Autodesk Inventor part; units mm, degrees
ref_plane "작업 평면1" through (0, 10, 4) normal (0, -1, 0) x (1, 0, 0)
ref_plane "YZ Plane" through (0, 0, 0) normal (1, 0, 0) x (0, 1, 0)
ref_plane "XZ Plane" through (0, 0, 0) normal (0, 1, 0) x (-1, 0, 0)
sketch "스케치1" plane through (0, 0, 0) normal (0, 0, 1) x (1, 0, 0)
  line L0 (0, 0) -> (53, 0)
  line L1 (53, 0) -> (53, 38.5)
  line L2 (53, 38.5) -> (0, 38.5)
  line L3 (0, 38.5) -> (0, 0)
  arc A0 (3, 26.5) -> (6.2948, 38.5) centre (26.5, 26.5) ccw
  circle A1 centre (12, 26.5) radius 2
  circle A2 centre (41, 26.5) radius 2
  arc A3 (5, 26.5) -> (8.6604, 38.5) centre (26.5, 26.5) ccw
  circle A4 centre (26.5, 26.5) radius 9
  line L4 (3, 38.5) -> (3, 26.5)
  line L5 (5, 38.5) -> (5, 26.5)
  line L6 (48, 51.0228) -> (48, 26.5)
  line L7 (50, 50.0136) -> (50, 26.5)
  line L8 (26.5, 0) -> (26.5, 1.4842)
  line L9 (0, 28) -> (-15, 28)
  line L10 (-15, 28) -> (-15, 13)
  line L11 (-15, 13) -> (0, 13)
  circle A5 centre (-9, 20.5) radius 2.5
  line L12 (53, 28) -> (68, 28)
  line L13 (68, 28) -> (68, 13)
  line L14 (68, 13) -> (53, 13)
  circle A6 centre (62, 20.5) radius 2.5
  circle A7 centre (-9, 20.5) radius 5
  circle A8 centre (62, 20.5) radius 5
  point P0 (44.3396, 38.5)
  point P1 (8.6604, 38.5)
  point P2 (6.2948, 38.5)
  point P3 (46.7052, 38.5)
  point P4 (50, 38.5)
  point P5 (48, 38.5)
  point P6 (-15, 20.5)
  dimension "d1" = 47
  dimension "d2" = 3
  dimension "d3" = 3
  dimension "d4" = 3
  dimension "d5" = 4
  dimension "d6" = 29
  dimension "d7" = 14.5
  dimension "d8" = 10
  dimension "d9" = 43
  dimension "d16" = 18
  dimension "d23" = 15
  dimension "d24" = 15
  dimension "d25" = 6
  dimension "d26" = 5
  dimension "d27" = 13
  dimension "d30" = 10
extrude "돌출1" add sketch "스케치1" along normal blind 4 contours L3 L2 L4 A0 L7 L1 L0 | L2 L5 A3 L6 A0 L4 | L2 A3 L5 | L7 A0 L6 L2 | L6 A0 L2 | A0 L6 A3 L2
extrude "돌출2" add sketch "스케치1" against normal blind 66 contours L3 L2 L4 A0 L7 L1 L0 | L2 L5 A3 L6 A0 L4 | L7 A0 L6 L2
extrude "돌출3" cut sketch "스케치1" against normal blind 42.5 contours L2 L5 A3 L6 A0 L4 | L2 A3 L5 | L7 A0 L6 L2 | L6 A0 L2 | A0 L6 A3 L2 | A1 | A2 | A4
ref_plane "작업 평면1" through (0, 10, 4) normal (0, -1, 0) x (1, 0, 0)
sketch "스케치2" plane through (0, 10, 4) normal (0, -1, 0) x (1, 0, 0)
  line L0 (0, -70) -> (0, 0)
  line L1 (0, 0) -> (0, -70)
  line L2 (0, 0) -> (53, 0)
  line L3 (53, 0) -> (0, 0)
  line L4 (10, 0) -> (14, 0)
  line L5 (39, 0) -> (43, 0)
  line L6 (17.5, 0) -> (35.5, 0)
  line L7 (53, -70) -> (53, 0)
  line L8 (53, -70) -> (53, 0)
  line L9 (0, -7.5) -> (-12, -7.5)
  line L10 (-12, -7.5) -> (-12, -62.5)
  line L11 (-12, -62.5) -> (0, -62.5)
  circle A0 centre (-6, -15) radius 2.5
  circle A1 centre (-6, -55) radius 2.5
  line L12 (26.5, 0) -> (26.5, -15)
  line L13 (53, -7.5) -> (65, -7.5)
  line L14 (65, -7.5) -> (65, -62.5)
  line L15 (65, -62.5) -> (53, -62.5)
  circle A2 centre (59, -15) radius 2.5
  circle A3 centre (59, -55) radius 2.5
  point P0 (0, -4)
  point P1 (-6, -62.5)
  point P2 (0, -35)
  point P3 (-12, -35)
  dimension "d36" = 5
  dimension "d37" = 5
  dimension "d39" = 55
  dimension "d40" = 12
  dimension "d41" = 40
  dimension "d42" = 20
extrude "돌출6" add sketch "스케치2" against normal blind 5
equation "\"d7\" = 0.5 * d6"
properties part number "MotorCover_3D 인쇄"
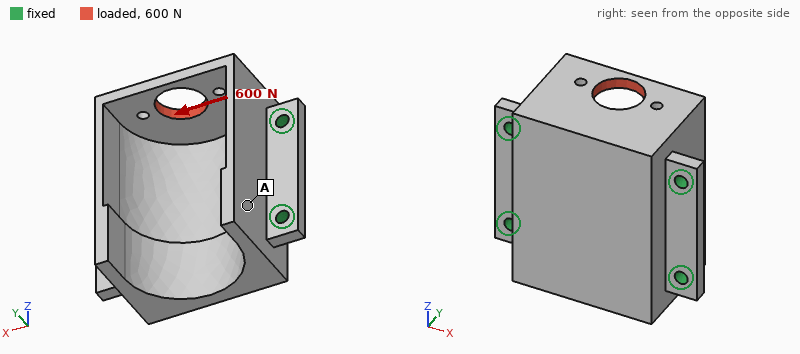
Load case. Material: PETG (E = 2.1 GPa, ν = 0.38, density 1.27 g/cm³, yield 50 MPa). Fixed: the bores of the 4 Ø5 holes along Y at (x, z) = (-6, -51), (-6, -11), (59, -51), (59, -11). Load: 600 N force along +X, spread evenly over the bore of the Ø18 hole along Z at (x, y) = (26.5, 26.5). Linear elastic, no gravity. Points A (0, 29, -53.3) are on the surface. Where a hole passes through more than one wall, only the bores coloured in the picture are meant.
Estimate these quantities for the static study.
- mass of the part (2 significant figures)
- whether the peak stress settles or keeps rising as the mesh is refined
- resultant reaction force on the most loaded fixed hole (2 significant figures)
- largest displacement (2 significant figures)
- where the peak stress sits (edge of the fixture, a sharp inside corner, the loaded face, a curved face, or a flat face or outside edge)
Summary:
74 g
keeps rising
380 N
0.34 mm
edge of the fixture
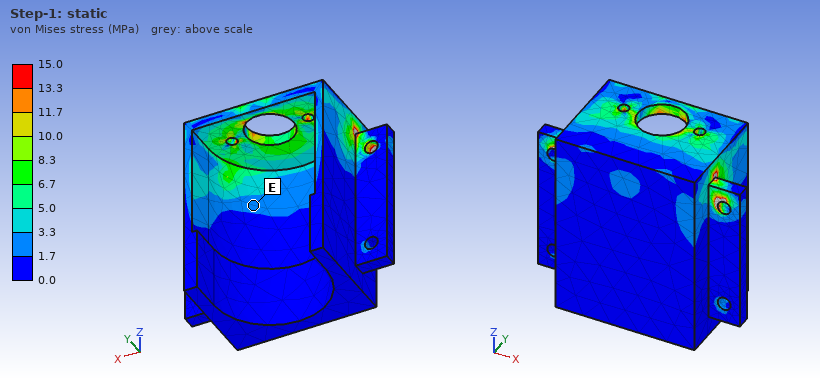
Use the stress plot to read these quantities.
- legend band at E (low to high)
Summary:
1.7 to 3.3 MPa
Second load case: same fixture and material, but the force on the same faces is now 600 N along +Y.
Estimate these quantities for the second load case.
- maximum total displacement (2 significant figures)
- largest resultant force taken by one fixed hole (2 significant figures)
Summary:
0.39 mm
420 N
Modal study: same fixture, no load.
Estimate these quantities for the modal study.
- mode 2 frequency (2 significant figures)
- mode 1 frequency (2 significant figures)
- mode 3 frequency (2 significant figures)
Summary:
1800 Hz
1700 Hz
1900 Hz
